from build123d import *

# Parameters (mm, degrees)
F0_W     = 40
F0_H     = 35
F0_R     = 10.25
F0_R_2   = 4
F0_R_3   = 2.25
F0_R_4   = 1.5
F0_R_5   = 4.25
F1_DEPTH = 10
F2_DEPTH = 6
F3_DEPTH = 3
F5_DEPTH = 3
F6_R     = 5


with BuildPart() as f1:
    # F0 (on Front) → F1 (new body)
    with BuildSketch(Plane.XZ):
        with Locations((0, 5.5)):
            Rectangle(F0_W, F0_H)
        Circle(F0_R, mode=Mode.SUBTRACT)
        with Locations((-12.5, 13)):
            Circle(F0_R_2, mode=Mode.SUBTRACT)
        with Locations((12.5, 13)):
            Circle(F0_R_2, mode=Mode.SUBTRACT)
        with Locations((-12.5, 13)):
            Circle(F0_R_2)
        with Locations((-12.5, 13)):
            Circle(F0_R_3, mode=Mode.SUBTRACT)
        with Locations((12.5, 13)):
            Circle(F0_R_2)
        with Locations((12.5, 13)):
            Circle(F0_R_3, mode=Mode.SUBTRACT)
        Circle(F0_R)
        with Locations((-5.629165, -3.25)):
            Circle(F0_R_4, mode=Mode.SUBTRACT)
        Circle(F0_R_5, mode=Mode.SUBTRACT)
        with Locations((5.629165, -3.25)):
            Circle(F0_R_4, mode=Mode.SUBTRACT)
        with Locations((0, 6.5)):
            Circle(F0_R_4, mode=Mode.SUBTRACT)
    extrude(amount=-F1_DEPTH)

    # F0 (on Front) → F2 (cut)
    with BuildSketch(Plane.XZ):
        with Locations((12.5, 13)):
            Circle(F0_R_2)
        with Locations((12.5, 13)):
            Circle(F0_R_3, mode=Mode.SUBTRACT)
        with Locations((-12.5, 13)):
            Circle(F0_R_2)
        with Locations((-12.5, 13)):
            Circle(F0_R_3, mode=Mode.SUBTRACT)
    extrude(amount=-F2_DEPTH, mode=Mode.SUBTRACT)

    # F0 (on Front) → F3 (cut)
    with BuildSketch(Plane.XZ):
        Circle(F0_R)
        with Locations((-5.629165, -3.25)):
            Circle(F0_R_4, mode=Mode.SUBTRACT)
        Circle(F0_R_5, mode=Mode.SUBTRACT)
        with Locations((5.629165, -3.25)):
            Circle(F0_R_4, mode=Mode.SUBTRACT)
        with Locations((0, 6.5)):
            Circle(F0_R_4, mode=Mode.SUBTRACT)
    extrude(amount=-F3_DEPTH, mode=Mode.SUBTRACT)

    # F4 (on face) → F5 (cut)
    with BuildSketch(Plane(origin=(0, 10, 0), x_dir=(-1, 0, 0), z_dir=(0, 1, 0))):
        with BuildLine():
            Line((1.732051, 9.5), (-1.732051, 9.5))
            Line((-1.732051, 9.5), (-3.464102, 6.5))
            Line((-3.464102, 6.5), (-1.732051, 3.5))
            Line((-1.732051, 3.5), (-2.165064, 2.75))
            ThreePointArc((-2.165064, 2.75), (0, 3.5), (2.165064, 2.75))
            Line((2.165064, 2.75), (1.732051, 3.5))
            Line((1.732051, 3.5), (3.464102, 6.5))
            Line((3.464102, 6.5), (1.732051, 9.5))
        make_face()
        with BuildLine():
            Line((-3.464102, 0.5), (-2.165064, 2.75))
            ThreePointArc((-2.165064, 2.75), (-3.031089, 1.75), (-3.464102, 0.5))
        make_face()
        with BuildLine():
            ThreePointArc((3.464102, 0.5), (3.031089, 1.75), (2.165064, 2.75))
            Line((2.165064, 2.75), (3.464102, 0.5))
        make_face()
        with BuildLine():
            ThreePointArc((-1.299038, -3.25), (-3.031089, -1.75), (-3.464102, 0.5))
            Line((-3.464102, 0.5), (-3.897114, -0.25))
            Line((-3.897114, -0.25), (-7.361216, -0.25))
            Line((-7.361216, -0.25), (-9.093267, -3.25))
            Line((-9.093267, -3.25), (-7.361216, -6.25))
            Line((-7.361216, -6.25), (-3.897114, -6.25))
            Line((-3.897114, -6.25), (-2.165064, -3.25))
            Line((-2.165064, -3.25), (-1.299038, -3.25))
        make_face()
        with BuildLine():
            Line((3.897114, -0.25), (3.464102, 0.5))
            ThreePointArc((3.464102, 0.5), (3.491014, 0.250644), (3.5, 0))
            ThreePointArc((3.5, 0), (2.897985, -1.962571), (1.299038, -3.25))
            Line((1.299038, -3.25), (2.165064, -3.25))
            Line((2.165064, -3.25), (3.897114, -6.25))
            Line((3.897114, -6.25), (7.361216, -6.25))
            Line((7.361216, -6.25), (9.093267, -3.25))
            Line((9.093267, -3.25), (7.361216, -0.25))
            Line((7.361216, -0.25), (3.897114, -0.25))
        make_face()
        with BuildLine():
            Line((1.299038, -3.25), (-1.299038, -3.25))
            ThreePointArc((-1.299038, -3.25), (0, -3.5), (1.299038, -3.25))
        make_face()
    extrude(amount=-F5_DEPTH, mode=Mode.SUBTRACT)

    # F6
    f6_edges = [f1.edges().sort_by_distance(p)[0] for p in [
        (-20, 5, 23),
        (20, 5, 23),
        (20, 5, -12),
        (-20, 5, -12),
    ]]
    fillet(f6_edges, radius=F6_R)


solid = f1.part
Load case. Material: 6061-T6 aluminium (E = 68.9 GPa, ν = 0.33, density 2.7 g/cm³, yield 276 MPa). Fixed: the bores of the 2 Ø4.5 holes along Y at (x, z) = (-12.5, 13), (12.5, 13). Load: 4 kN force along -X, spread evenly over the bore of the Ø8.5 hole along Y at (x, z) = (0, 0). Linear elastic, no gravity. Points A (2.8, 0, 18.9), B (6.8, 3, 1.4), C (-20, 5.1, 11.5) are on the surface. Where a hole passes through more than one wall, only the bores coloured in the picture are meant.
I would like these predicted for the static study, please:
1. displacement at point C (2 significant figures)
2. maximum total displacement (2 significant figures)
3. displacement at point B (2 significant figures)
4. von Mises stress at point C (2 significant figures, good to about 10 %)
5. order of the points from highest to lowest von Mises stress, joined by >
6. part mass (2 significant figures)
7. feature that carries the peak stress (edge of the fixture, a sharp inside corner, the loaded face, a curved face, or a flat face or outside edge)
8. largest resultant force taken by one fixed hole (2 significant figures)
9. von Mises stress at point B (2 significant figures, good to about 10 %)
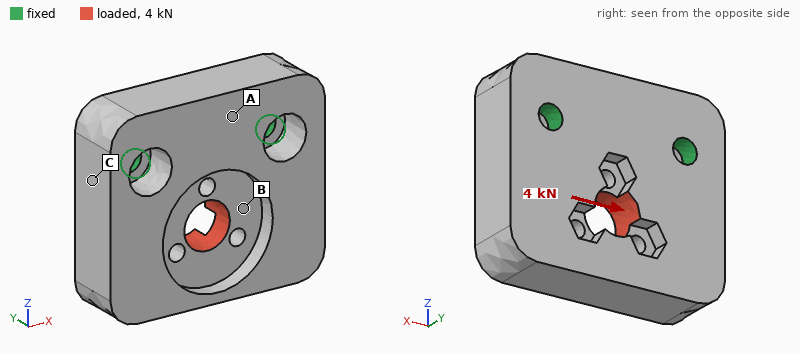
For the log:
8.2 µm
31 µm
15 µm
25 MPa
B > C > A
31 g
a curved face
2.7 kN
44 MPa
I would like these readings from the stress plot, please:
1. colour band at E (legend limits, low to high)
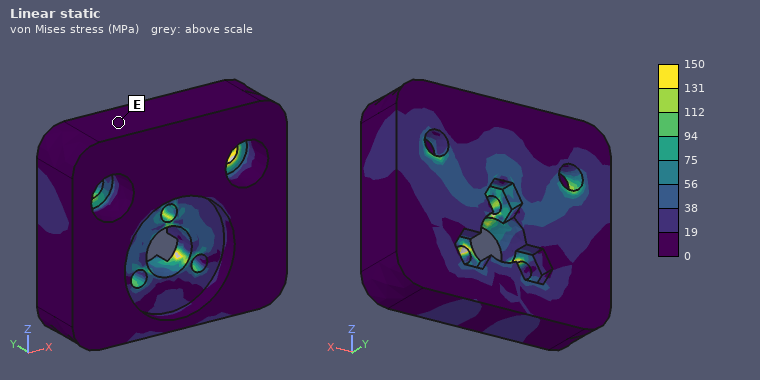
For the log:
0 to 19 MPa
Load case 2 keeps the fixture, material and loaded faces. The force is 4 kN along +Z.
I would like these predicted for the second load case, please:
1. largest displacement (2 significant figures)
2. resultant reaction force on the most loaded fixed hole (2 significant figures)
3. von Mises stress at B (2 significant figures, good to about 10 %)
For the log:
27 µm
2.0 kN
28 MPa
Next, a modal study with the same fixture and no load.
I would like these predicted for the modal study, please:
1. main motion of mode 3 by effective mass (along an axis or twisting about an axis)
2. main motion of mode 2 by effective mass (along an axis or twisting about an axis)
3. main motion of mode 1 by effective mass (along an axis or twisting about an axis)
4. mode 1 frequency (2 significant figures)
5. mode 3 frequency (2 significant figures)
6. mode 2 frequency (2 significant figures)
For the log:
along X
twisting about Z
along Y
5900 Hz
16 kHz
12 kHz
